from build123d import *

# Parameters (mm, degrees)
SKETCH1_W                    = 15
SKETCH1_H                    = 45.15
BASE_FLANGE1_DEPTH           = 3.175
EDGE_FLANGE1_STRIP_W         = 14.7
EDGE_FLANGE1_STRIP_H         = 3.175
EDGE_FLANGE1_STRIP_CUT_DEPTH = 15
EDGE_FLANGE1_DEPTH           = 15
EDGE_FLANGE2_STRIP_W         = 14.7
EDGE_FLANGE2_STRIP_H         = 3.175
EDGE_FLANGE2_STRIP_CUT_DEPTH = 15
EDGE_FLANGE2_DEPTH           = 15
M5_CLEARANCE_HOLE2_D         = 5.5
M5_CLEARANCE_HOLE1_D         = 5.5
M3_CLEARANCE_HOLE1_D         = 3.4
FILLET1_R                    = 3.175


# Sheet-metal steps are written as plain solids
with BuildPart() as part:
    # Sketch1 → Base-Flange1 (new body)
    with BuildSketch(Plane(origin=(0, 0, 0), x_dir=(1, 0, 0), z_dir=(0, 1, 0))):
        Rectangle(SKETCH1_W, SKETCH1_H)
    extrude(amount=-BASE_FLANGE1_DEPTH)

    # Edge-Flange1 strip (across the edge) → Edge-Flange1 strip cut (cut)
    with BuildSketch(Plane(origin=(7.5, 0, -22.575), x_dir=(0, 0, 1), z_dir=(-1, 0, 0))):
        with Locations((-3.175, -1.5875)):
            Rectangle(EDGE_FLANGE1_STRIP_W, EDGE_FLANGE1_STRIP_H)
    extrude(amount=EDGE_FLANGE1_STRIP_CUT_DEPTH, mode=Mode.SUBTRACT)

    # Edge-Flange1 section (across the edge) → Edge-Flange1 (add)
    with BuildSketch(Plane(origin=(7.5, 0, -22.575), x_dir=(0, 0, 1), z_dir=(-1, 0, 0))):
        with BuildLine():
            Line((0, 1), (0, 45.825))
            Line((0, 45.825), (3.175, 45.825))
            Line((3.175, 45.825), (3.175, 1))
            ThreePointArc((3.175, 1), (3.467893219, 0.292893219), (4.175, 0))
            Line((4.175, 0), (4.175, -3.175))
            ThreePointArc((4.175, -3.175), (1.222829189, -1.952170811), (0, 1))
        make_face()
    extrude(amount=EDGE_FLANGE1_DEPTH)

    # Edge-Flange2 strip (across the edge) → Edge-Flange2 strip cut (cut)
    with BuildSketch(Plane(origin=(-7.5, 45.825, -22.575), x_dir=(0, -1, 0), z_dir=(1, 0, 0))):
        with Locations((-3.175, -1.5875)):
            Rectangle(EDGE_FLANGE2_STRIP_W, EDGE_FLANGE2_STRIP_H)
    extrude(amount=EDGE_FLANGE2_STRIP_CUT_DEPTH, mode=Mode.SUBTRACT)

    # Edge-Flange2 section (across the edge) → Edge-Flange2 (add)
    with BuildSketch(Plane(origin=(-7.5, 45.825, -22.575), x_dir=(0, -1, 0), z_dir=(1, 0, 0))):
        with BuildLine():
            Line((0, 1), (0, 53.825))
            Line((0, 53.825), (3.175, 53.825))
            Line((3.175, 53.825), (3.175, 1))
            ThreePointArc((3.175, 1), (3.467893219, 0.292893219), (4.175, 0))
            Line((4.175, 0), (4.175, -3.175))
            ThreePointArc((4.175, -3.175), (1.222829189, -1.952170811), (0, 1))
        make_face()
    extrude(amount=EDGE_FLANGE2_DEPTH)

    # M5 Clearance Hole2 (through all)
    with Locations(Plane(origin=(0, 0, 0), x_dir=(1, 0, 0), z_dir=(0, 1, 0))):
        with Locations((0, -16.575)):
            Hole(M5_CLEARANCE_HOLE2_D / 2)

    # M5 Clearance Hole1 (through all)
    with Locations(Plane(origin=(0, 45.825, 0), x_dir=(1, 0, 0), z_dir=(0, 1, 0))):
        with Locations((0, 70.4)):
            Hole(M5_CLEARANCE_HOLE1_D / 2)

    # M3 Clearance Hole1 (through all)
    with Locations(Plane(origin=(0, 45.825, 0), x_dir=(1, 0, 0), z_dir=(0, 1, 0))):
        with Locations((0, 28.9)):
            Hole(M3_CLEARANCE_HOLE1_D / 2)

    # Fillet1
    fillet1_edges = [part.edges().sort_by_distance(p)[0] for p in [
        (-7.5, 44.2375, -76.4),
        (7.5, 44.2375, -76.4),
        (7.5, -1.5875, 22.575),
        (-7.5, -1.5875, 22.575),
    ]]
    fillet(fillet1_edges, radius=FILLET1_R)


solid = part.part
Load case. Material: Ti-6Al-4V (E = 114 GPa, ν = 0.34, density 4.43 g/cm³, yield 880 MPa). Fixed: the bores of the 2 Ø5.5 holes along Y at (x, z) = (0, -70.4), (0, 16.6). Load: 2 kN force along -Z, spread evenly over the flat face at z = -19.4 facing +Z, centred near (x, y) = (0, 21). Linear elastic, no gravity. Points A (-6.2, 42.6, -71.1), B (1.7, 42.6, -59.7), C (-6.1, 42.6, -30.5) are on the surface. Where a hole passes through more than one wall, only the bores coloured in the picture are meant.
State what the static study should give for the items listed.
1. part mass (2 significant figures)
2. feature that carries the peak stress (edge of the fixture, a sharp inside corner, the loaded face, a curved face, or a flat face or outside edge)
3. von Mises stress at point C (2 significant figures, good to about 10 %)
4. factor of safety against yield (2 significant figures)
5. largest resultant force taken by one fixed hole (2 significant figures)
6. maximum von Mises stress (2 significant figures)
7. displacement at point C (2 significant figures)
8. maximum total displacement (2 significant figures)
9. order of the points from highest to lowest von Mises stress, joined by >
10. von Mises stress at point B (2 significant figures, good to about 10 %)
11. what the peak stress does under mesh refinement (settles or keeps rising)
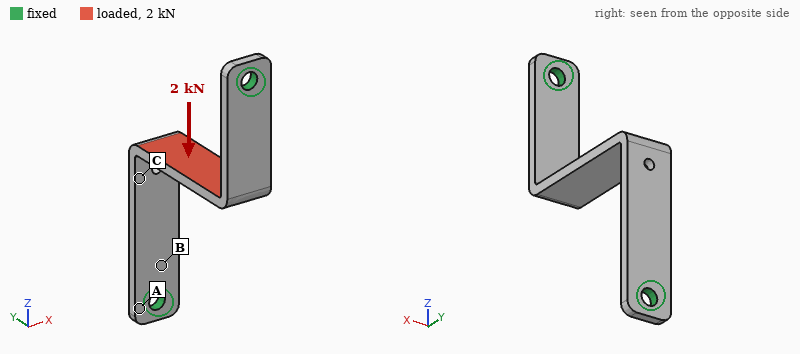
29 g
the loaded face
170 MPa
2.3
1.0 kN
380 MPa
0.32 mm
0.70 mm
C > B > A
94 MPa
settles
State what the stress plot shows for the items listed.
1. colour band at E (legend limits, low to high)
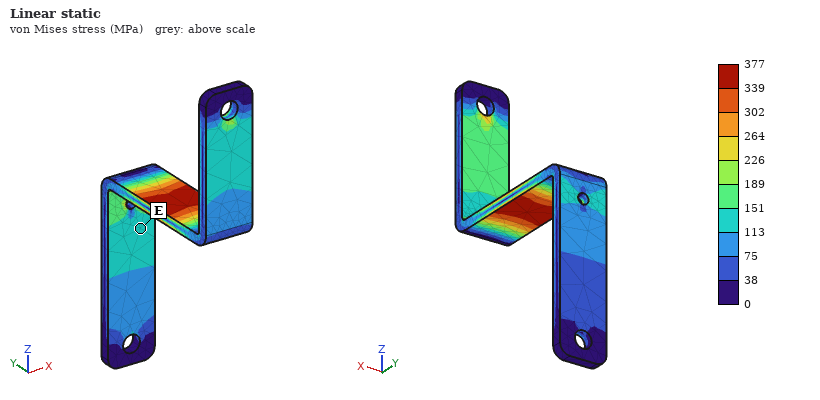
113 to 151 MPa
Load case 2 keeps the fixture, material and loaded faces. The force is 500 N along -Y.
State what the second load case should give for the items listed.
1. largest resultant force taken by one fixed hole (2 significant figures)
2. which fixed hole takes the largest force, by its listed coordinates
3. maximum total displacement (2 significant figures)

360 N
(0, 16.6)
0.63 mm
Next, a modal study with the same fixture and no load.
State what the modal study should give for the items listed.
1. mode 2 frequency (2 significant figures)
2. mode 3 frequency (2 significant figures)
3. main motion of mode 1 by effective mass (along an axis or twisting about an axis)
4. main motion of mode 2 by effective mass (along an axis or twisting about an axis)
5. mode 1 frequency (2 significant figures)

2900 Hz
4600 Hz
along Y
along X
1200 Hz
